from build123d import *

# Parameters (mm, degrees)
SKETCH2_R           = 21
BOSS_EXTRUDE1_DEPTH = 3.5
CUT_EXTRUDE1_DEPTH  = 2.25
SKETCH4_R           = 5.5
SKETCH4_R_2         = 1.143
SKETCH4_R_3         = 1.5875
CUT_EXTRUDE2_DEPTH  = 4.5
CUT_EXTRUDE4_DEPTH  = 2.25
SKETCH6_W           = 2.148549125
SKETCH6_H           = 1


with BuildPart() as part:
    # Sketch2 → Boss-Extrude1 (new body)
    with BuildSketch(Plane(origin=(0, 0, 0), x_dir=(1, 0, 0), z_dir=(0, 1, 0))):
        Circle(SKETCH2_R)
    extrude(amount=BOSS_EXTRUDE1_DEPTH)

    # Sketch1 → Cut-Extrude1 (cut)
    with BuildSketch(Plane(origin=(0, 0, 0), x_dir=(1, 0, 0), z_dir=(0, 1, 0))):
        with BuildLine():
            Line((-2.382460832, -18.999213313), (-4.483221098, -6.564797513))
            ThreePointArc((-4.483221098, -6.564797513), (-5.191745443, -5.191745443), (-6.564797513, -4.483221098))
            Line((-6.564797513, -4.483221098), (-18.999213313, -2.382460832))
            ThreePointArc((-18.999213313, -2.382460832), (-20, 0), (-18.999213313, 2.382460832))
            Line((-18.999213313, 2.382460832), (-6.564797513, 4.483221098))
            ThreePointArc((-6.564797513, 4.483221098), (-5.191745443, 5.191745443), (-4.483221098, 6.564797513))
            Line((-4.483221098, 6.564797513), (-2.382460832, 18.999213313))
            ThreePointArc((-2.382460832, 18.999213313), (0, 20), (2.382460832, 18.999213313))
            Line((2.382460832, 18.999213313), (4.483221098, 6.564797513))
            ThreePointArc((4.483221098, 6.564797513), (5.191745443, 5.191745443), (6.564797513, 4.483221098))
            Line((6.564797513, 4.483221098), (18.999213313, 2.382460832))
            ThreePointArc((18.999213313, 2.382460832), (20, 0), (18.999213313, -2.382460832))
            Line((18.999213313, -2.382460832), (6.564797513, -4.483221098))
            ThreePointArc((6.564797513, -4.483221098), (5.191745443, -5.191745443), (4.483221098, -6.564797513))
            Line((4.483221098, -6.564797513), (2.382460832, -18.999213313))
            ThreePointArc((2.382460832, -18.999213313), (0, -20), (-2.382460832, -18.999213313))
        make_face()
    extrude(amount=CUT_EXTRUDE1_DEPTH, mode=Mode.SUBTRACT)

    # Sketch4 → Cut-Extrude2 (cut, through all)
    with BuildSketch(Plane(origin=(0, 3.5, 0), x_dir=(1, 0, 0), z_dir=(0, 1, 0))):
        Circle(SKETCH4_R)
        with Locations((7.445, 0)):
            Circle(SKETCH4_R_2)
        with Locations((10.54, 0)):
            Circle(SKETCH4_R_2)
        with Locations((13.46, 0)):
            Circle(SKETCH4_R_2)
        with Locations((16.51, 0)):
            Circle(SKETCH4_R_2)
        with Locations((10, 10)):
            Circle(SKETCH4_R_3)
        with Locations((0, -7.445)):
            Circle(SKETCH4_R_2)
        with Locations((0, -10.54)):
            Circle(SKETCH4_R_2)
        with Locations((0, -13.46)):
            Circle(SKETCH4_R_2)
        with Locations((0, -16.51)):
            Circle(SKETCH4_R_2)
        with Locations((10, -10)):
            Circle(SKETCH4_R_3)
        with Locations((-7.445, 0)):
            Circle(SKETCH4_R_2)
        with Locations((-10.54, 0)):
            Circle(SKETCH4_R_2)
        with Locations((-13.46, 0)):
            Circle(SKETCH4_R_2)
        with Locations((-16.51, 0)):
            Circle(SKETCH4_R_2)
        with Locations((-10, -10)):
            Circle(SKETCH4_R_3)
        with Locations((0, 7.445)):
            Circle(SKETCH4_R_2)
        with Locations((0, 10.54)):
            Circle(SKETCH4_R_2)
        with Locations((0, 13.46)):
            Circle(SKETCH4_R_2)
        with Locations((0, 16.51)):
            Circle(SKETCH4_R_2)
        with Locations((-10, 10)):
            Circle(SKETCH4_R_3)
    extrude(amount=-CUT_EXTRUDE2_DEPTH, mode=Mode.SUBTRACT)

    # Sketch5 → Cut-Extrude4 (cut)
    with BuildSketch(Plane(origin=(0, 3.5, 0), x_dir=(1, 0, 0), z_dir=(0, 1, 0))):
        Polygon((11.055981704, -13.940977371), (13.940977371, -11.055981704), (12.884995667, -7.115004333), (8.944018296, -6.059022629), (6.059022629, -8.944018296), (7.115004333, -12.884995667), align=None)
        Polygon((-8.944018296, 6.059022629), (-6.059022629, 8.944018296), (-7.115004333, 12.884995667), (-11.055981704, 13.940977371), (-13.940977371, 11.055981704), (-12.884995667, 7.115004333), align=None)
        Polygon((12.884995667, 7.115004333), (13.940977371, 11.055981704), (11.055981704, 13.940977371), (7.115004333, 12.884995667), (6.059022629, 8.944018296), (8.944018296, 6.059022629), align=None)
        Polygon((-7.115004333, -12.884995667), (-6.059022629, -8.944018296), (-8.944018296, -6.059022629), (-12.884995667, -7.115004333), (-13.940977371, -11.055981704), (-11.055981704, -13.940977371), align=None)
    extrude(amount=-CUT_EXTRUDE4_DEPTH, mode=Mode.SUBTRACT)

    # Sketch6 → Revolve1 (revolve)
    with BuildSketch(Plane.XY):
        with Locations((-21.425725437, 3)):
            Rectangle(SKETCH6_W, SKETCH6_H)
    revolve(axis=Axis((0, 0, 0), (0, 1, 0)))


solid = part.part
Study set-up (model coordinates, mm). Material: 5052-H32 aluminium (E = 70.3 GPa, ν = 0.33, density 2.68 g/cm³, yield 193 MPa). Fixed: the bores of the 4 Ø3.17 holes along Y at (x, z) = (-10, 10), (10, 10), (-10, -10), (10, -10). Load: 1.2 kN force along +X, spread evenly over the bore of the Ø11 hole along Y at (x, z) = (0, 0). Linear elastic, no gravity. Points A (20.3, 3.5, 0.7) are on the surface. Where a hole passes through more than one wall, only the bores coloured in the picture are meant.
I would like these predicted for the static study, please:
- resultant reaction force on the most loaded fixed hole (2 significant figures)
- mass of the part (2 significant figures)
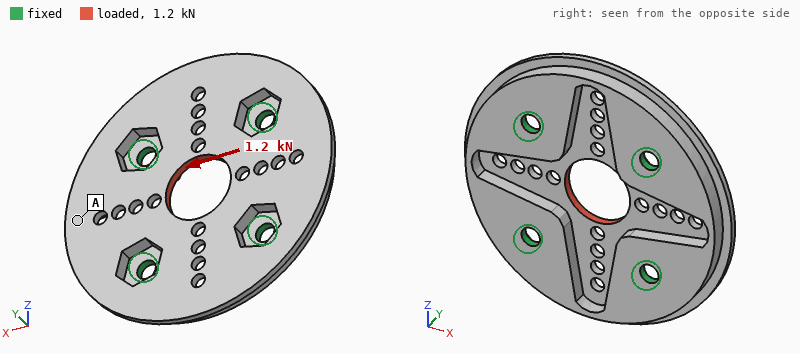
300 N
8.8 g
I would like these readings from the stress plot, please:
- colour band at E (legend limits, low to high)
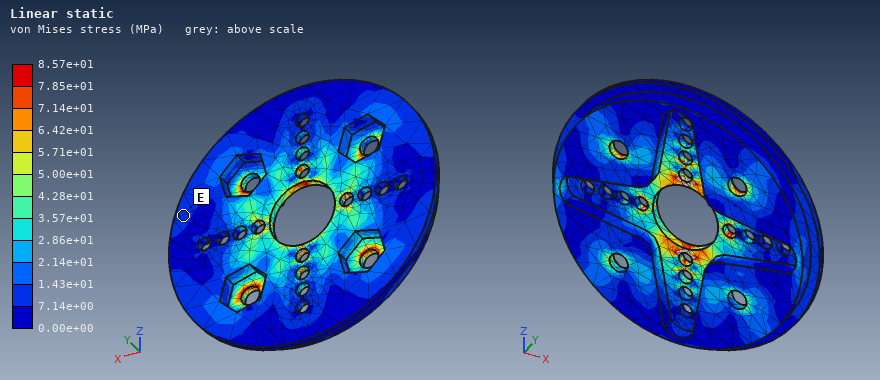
7.14e+00 to 1.43e+01 MPa
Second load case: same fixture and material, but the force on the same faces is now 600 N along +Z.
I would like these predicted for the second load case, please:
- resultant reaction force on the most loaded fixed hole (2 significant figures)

150 N
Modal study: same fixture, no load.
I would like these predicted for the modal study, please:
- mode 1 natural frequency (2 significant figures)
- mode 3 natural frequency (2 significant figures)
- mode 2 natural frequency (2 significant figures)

12 kHz
14 kHz
14 kHz
